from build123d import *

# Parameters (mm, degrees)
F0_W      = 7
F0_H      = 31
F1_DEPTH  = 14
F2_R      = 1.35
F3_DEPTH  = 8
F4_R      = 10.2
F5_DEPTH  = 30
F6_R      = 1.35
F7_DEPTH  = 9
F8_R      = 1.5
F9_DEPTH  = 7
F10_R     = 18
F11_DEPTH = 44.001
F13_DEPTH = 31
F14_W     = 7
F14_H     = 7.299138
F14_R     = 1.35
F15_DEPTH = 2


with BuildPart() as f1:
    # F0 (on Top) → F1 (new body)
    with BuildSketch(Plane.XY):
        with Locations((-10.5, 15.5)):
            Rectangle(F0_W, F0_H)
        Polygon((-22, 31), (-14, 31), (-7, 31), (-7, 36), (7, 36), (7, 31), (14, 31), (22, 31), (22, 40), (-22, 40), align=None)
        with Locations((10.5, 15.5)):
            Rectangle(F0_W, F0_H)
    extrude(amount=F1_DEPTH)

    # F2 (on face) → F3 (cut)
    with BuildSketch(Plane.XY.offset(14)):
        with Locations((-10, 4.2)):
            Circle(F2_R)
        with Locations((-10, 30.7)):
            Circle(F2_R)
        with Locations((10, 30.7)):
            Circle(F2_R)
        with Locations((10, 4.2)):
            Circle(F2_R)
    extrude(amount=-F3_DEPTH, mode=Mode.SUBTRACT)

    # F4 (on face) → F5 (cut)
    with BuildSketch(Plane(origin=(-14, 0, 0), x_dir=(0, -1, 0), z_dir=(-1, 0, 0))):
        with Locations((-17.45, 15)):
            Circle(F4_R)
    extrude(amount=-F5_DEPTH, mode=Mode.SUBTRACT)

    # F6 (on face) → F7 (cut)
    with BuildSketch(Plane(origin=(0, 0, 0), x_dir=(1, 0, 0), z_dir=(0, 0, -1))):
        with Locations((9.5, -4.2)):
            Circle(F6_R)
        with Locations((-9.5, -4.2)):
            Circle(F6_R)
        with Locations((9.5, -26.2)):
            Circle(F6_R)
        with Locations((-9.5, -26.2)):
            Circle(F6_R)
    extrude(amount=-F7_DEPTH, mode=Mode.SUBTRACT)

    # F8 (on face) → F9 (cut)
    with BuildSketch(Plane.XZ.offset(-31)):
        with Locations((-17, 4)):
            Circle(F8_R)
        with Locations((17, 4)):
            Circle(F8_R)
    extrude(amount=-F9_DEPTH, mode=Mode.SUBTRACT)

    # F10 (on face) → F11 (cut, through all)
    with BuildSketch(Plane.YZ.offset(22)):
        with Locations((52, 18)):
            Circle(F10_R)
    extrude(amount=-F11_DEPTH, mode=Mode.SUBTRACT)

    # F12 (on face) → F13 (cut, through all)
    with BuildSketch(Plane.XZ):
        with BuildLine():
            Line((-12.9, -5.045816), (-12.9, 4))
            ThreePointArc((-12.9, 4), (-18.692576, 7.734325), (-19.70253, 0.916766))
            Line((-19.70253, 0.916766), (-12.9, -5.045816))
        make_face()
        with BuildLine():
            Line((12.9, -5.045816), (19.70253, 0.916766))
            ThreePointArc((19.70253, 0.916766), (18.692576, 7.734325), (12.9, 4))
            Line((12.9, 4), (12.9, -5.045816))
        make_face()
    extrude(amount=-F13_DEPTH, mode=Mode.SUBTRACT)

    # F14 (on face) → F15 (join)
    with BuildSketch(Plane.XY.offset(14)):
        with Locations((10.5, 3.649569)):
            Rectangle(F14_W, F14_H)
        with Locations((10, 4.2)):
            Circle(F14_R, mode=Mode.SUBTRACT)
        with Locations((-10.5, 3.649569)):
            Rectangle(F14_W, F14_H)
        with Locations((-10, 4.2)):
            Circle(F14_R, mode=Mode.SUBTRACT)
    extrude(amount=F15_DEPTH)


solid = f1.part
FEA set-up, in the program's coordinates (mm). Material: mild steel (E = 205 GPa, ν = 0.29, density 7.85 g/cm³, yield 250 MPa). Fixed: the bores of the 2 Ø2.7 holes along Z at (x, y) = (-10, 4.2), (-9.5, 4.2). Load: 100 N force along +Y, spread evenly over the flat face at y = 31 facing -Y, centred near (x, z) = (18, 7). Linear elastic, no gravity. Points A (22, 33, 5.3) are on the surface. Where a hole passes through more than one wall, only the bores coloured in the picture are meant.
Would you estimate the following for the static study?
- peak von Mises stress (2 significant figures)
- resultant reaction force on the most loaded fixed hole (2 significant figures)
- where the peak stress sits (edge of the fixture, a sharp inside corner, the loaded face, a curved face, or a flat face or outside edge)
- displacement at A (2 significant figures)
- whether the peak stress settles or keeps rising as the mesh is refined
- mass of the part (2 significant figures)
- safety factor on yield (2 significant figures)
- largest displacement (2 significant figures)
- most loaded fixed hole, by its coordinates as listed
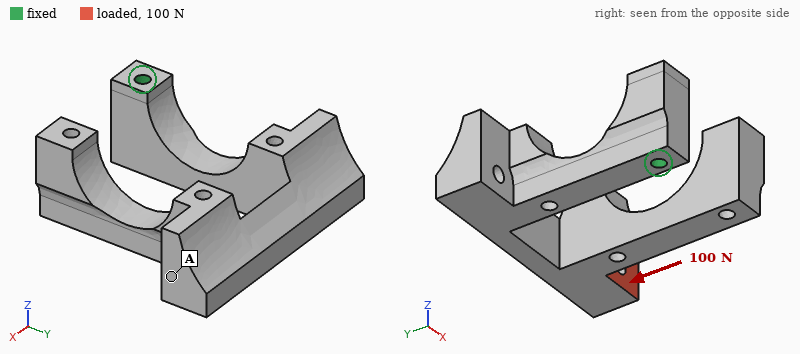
170 MPa
150 N
a curved face
0.24 mm
settles
52 g
1.5
0.31 mm
(-9.5, 4.2)
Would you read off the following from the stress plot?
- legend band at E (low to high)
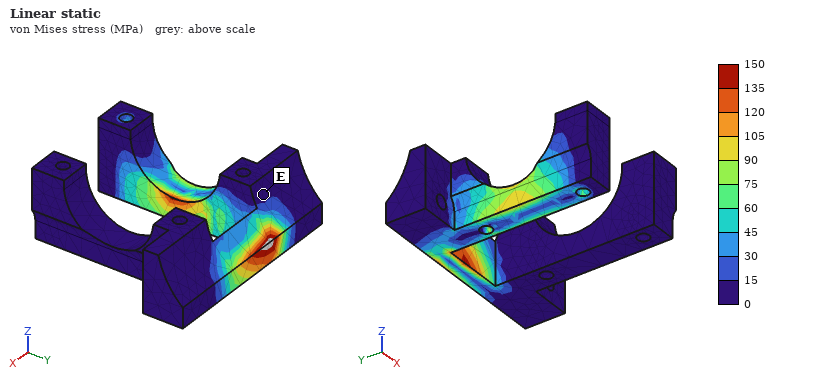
0 to 15 MPa
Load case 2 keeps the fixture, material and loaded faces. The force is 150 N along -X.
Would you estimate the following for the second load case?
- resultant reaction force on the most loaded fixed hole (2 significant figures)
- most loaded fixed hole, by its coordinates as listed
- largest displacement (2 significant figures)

190 N
(-9.5, 4.2)
84 µm
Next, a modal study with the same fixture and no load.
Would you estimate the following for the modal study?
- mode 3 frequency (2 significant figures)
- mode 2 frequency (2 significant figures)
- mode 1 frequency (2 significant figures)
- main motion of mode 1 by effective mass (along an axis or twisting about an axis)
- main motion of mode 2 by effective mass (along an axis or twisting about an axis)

1200 Hz
760 Hz
680 Hz
along Y
along Z
